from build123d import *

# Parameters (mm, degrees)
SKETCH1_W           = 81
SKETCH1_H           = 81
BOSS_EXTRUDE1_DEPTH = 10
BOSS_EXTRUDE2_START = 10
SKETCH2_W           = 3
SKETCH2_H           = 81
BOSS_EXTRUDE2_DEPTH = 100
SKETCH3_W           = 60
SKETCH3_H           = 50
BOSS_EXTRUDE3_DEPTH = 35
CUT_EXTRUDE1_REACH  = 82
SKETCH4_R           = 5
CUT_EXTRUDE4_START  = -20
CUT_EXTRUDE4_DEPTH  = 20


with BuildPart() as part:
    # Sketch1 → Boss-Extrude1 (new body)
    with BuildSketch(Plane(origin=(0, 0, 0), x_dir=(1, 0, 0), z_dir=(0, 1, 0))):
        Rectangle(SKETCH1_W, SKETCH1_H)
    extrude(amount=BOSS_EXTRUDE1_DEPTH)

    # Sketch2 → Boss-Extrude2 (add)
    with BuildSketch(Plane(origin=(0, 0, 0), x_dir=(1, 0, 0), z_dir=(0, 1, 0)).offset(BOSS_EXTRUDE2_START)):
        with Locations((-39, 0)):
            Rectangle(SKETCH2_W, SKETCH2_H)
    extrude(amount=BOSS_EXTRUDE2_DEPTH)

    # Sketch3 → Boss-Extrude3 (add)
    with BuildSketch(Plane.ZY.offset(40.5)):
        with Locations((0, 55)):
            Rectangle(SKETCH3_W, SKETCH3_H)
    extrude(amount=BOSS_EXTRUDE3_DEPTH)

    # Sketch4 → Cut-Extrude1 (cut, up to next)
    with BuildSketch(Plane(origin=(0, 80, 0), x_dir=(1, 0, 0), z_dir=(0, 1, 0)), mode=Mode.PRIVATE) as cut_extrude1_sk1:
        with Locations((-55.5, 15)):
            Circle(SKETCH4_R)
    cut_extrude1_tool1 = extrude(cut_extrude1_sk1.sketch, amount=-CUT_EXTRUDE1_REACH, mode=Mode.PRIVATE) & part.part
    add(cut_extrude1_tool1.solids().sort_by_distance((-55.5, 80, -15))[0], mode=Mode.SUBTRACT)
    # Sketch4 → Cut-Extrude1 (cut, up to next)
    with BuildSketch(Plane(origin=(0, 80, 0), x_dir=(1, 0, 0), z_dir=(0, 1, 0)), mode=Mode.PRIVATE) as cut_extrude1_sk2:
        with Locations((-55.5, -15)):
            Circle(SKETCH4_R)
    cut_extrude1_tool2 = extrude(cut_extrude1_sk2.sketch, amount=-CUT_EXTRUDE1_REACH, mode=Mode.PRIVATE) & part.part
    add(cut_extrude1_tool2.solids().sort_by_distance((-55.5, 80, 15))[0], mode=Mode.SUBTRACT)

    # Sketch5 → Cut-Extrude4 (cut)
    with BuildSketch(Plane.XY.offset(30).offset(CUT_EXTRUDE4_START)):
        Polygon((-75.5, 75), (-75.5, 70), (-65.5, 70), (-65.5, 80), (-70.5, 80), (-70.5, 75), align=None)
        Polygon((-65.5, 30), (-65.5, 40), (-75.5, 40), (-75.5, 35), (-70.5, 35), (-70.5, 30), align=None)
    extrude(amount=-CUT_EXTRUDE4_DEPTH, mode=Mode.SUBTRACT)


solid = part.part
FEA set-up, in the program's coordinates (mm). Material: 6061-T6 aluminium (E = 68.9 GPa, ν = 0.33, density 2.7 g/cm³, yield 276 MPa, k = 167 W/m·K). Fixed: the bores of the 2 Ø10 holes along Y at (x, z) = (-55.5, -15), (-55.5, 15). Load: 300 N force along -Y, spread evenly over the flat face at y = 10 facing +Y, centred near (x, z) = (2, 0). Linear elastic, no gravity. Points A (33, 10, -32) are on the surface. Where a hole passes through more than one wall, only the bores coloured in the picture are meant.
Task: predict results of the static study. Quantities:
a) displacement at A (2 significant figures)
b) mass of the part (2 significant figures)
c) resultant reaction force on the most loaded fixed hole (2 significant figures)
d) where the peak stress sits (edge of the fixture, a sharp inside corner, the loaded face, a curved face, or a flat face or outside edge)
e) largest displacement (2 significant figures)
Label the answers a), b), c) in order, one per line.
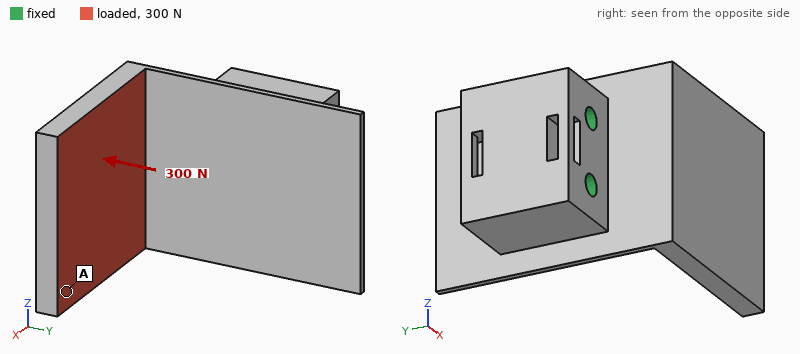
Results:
a) 1.4 mm
b) 500 g
c) 150 N
d) a flat face or outside edge
e) 1.6 mm
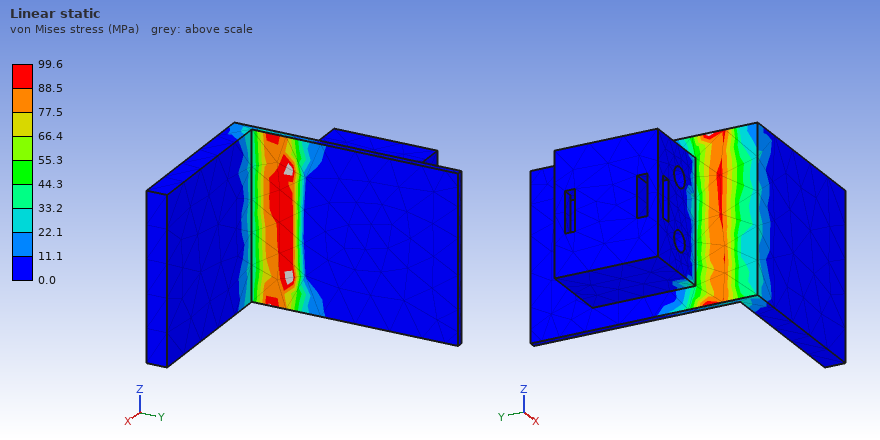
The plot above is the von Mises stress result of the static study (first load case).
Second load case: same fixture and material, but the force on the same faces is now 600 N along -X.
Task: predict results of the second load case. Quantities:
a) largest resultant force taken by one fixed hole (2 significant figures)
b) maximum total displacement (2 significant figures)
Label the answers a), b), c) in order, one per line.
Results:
a) 300 N
b) 0.82 mm
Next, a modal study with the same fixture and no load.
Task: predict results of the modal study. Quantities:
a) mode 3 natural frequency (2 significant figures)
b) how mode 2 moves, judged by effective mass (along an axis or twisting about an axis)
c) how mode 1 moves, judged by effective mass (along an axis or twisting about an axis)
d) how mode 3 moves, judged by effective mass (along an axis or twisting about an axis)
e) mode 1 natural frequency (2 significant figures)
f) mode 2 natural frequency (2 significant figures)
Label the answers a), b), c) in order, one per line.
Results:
a) 1400 Hz
b) along Z
c) along Y
d) along X
e) 190 Hz
f) 610 Hz
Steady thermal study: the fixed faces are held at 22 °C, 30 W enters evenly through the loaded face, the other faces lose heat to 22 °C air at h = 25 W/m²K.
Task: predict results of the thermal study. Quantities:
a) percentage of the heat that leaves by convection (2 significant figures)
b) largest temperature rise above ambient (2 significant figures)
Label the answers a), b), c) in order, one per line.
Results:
a) 21 %
b) 24 K
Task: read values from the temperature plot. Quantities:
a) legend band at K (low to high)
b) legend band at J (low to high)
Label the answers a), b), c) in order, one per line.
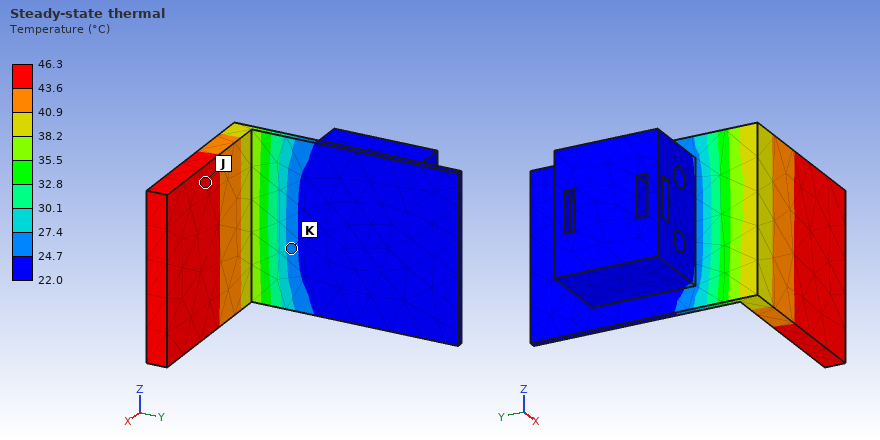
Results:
a) 24.7 to 27.4 °C
b) 43.6 to 46.3 °C
